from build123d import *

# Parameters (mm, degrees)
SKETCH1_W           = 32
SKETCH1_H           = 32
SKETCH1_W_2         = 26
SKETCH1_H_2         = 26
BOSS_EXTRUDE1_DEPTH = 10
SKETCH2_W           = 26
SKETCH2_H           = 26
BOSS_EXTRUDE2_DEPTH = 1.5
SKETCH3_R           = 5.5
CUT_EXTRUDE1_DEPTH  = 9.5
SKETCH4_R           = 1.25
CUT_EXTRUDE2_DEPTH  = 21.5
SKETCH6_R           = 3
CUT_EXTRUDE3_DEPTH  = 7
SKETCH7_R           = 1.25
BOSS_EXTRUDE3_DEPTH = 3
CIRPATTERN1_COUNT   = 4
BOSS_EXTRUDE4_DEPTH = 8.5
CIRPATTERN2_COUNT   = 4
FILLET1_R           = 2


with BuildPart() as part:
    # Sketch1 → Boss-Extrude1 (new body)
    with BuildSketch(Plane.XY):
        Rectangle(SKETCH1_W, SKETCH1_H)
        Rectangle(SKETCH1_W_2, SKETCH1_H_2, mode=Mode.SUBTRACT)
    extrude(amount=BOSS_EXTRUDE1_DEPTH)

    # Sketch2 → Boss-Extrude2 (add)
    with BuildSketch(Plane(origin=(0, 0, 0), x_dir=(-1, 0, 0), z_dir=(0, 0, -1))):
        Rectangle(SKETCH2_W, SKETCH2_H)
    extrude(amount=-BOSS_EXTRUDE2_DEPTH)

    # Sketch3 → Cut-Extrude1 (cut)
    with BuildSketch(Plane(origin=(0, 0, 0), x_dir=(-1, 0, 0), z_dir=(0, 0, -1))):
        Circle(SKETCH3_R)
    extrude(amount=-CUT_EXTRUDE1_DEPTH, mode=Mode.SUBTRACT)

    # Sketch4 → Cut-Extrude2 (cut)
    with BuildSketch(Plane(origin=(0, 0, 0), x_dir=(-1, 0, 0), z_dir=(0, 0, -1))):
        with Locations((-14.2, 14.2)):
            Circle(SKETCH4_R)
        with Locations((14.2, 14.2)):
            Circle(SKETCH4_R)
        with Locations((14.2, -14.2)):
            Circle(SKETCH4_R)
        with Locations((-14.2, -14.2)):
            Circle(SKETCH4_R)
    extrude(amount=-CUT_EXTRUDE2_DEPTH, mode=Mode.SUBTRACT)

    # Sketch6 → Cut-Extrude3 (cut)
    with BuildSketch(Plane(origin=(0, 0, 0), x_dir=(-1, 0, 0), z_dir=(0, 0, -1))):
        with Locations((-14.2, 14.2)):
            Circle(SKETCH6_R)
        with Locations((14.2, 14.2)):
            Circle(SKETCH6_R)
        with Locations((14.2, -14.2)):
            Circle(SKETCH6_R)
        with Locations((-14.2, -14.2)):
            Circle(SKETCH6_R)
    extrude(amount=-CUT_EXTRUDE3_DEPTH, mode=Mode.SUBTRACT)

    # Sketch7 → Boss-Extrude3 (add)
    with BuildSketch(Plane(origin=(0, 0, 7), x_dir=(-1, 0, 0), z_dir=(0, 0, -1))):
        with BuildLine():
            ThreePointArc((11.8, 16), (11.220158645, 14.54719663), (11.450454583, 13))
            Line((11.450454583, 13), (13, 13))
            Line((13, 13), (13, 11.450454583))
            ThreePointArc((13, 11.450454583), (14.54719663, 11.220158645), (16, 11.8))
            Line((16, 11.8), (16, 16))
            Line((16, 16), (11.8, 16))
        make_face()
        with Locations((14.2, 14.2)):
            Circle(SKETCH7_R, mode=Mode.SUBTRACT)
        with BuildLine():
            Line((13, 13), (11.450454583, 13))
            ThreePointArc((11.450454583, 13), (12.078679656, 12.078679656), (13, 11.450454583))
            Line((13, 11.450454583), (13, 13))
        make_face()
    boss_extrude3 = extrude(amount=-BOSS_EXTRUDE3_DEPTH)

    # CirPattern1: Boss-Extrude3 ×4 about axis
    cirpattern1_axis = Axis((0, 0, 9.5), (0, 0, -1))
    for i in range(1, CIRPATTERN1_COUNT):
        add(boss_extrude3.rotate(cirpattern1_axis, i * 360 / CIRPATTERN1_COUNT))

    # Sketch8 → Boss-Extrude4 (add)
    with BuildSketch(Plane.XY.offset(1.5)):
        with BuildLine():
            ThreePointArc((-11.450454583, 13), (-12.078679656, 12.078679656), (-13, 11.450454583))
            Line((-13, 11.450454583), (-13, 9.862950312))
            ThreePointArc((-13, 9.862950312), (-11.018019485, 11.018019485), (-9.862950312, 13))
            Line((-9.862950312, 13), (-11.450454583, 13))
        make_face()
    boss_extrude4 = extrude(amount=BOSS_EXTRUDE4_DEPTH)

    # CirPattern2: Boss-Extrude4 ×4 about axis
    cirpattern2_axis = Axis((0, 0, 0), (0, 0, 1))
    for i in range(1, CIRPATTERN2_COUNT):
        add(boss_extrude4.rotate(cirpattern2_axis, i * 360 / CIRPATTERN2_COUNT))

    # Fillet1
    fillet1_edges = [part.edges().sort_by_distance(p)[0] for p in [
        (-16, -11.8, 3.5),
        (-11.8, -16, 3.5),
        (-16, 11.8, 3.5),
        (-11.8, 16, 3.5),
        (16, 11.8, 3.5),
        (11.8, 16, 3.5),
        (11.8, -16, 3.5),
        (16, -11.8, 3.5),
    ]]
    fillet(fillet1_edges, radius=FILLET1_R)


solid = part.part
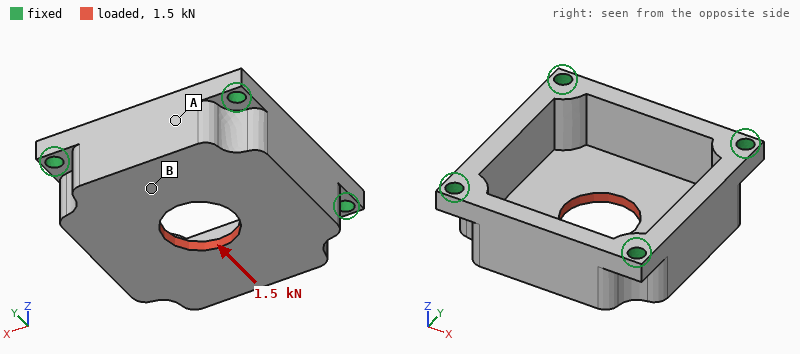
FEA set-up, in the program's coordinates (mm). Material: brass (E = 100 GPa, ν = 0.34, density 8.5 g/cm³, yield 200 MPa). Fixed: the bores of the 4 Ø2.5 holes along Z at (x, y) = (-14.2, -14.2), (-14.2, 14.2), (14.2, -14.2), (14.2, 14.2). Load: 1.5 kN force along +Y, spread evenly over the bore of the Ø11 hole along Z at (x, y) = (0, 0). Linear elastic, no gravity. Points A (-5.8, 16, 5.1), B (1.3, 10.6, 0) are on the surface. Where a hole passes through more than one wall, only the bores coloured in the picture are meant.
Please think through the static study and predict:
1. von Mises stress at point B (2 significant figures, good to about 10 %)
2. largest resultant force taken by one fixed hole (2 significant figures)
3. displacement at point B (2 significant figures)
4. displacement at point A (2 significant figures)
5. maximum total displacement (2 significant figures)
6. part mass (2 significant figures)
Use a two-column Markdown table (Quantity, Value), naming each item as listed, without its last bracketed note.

| Quantity | Value |
|---|---|
| von Mises stress at point B | 21 MPa |
| largest resultant force taken by one fixed hole | 430 N |
| displacement at point B | 9.8 µm |
| displacement at point A | 4.5 µm |
| maximum total displacement | 11 µm |
| part mass | 33 g |
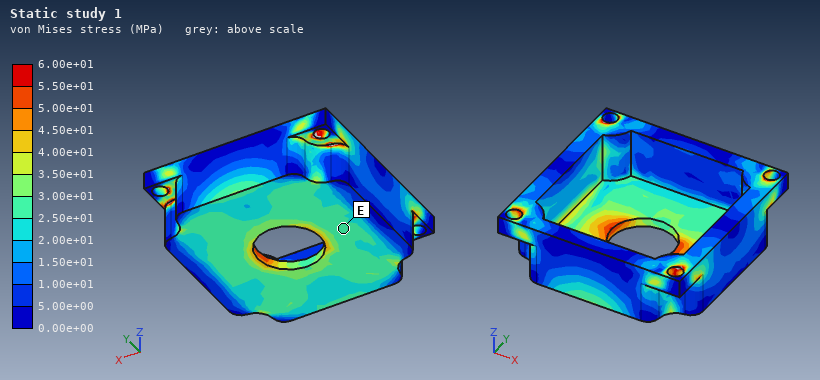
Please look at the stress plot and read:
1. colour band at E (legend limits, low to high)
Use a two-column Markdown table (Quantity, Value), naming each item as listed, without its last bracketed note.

| Quantity | Value |
|---|---|
| colour band at E | 2.50e+01 to 3.00e+01 MPa |
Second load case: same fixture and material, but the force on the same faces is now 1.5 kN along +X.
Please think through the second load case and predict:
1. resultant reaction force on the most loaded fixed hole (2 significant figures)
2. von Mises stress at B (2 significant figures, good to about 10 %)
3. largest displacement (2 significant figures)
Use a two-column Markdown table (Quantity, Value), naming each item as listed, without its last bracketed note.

| Quantity | Value |
|---|---|
| resultant reaction force on the most loaded fixed hole | 430 N |
| von Mises stress at B | 26 MPa |
| largest displacement | 11 µm |
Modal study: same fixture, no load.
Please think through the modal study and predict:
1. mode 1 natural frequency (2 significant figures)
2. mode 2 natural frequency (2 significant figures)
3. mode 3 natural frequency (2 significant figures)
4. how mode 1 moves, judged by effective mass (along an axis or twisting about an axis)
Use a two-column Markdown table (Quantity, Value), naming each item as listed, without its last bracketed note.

| Quantity | Value |
|---|---|
| mode 1 natural frequency | 12 kHz |
| mode 2 natural frequency | 16 kHz |
| mode 3 natural frequency | 17 kHz |
| how mode 1 moves, judged by effective mass | along Z |
